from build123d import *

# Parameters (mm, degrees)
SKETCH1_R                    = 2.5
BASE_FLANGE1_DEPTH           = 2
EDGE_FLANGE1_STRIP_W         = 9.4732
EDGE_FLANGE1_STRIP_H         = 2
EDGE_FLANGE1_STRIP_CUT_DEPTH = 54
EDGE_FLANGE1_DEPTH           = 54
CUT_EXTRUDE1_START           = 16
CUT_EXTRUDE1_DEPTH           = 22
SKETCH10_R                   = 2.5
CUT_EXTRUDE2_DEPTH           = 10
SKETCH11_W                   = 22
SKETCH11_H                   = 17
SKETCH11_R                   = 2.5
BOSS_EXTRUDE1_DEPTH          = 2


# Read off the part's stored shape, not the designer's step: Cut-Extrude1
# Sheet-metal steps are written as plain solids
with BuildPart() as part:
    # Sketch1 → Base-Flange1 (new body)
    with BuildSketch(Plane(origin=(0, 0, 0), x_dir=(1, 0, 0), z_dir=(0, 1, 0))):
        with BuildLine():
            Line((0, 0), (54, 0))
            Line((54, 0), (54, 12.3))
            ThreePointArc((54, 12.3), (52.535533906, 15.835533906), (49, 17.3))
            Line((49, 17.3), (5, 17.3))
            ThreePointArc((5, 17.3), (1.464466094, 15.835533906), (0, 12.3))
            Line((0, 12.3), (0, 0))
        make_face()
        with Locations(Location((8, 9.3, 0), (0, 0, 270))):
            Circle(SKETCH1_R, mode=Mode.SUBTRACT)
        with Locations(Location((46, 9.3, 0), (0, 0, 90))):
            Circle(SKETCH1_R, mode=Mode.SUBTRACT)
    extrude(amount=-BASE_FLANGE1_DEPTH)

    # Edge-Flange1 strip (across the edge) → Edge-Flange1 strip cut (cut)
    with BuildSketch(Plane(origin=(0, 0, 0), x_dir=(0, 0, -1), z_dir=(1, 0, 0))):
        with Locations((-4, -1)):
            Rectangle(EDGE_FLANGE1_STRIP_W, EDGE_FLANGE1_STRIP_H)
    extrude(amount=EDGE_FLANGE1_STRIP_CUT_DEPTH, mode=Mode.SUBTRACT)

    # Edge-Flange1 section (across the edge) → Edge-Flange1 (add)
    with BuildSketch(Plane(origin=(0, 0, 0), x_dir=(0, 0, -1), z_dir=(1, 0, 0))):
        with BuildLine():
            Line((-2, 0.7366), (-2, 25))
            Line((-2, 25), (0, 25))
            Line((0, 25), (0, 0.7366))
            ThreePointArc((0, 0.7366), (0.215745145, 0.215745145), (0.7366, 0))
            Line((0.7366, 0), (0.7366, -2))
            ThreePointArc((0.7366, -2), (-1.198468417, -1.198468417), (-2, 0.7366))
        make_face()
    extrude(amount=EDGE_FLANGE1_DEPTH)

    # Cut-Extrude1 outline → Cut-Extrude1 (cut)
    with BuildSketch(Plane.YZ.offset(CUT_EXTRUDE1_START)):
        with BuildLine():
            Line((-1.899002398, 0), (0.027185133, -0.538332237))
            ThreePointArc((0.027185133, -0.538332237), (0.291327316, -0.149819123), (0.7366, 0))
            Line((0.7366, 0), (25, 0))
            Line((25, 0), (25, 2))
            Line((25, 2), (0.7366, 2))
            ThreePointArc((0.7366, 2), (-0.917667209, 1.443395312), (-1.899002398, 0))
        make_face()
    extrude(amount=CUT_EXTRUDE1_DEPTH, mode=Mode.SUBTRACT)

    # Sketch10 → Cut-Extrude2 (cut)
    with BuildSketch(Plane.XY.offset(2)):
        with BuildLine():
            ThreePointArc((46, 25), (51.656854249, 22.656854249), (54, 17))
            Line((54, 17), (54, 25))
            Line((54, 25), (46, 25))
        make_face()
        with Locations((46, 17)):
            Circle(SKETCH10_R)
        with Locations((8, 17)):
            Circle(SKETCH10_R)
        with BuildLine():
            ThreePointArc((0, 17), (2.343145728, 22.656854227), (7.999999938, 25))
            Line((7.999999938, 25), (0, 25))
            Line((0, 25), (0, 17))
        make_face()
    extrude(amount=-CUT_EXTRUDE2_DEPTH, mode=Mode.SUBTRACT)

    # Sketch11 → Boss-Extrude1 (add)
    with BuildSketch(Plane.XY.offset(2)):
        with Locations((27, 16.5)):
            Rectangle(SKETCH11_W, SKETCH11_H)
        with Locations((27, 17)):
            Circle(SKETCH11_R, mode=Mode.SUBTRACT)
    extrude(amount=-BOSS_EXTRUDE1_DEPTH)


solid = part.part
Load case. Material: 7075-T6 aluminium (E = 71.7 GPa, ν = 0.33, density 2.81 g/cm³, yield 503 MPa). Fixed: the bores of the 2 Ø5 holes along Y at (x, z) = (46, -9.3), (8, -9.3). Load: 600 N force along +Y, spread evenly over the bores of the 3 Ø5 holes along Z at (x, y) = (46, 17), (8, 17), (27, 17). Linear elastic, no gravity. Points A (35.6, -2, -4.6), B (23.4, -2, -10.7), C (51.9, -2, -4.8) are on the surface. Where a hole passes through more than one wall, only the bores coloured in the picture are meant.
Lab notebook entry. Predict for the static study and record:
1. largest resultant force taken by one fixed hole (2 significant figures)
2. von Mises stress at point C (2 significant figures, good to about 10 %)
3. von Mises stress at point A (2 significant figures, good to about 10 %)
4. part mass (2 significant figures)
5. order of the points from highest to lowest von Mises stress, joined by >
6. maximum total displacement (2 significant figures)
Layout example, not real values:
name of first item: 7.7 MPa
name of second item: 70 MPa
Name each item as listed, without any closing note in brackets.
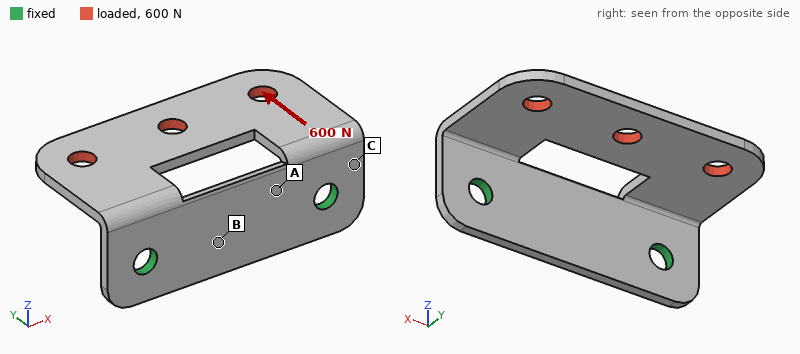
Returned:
largest resultant force taken by one fixed hole: 300 N
von Mises stress at point C: 110 MPa
von Mises stress at point A: 46 MPa
part mass: 11 g
order of the points from highest to lowest von Mises stress, joined by >: C > A > B
maximum total displacement: 0.36 mm
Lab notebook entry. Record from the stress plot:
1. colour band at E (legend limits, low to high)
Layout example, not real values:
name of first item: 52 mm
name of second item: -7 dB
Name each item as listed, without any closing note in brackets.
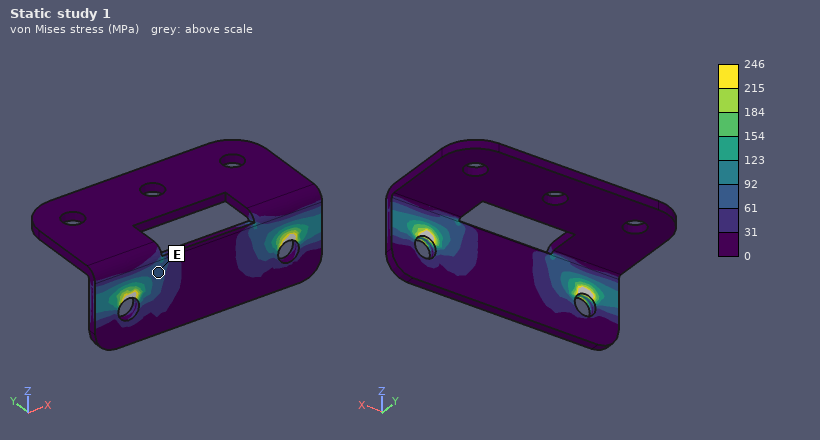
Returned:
colour band at E: 61 to 92 MPa
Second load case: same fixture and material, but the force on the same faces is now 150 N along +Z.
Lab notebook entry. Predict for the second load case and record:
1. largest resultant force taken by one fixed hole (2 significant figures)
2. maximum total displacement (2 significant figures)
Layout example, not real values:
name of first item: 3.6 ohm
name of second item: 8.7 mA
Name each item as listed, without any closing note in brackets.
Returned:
largest resultant force taken by one fixed hole: 76 N
maximum total displacement: 0.66 mm
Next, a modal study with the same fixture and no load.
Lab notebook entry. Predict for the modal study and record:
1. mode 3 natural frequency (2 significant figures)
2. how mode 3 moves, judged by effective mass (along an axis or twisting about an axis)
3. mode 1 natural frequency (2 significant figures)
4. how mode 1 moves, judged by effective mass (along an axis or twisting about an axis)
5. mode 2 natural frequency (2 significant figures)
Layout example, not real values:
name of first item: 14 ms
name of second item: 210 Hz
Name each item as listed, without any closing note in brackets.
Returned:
mode 3 natural frequency: 5800 Hz
how mode 3 moves, judged by effective mass: along Y
mode 1 natural frequency: 1400 Hz
how mode 1 moves, judged by effective mass: along Z
mode 2 natural frequency: 2800 Hz
